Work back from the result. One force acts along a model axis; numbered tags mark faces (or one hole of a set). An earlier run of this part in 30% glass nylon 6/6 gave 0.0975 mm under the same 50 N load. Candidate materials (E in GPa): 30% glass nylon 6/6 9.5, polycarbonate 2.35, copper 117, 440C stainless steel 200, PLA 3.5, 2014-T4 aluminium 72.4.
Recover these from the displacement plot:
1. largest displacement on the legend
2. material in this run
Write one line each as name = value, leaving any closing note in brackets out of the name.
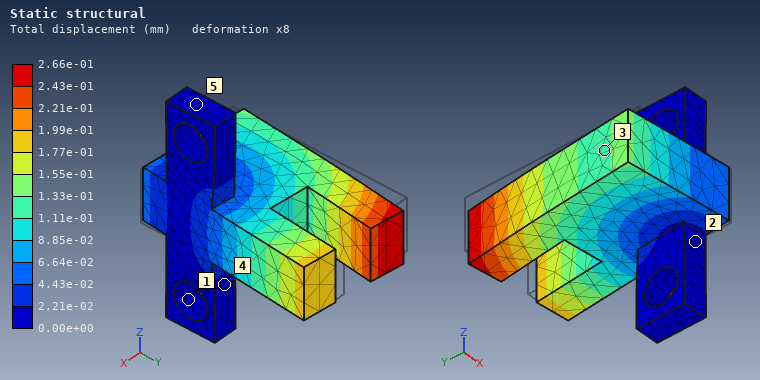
largest displacement on the legend = 2.66e-01 mm
material in this run = PLA
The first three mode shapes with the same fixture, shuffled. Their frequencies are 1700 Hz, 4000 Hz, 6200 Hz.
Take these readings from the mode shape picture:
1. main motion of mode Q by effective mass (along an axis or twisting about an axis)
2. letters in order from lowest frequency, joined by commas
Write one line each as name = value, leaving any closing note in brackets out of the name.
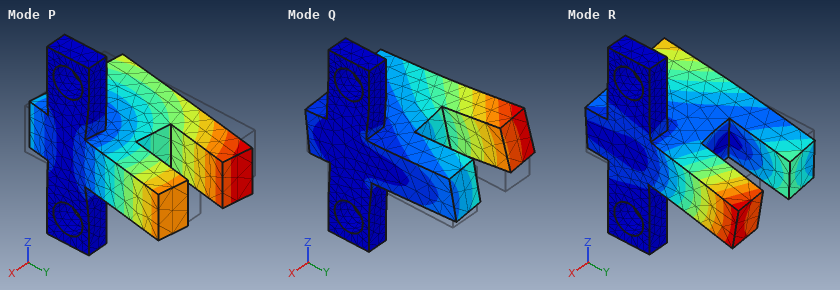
main motion of mode Q by effective mass = along Z
letters in order from lowest frequency, joined by commas = P, Q, R
